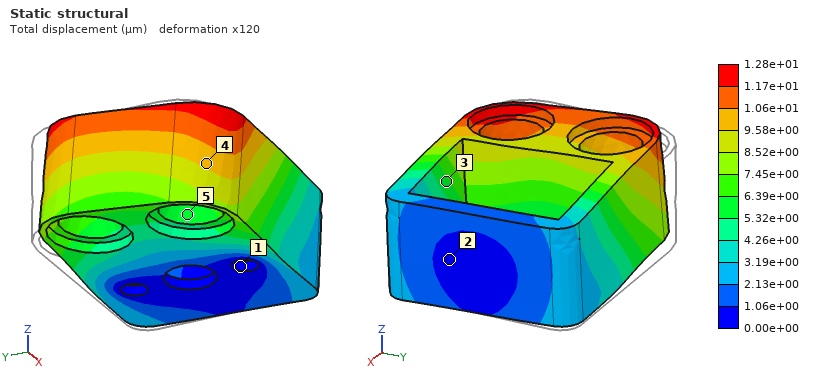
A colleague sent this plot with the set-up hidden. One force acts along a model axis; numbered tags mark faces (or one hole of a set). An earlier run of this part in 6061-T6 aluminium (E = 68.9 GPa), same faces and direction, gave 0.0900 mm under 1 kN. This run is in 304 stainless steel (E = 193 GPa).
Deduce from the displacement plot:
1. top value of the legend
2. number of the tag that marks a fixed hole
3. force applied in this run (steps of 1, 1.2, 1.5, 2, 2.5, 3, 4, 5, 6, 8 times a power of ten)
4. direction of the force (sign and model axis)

1.28e+01 µm
1
400 N
-Y
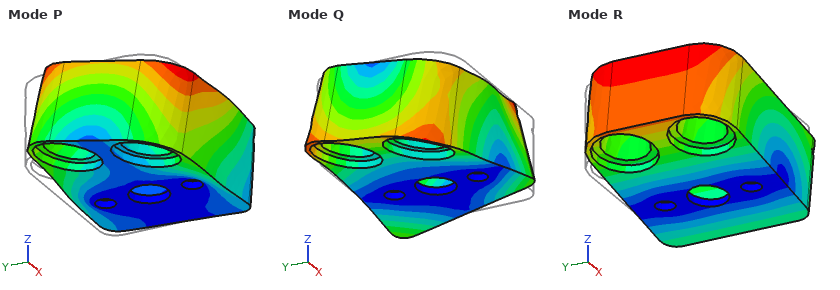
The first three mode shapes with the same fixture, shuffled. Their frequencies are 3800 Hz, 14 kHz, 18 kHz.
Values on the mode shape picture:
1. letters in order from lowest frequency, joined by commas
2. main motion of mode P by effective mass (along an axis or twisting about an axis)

R, P, Q
along Y
